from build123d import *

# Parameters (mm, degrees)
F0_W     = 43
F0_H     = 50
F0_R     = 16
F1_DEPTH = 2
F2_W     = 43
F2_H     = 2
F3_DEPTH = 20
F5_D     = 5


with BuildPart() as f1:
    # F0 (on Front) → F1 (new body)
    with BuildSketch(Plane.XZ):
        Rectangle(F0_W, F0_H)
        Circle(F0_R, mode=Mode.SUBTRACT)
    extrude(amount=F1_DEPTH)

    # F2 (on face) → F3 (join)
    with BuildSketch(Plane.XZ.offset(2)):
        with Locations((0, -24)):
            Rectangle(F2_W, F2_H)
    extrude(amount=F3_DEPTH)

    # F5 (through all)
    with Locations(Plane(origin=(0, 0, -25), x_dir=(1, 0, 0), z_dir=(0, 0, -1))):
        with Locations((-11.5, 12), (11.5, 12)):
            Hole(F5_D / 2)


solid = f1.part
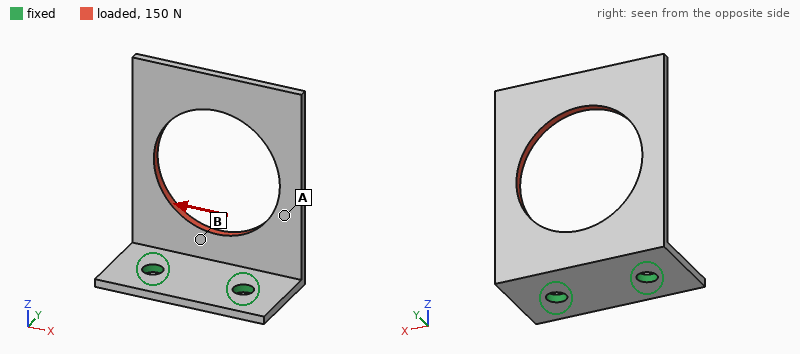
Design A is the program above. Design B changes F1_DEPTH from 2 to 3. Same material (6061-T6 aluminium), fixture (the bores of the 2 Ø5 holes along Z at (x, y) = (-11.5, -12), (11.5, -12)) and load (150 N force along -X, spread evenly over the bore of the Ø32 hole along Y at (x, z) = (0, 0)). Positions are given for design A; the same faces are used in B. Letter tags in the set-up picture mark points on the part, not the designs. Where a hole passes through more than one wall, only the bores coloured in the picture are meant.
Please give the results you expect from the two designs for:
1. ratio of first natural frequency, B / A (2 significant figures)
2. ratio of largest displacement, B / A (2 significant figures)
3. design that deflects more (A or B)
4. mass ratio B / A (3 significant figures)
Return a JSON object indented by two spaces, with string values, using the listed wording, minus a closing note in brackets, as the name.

{
  "ratio of first natural frequency, B / A": "1.2",
  "ratio of largest displacement, B / A": "0.64",
  "design that deflects more": "A",
  "mass ratio B / A": "1.29"
}
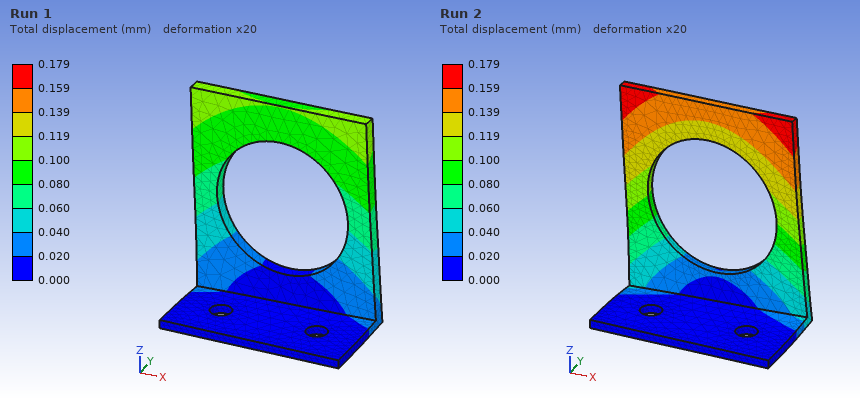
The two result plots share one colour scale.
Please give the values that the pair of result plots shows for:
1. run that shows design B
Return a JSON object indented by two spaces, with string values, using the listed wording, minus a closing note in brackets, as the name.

{
  "run that shows design B": "Run 1"
}
